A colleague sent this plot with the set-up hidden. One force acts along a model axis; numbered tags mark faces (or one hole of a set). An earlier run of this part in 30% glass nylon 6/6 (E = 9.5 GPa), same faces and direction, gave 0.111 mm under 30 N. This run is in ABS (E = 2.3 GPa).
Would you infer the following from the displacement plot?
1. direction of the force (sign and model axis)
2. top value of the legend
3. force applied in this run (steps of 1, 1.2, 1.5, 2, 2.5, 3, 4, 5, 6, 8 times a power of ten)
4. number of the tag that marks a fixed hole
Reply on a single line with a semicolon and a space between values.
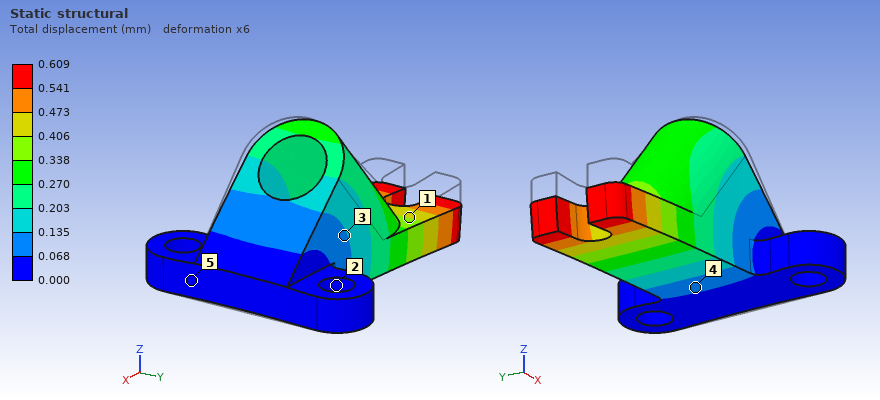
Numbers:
-Z; 0.609 mm; 40 N; 2
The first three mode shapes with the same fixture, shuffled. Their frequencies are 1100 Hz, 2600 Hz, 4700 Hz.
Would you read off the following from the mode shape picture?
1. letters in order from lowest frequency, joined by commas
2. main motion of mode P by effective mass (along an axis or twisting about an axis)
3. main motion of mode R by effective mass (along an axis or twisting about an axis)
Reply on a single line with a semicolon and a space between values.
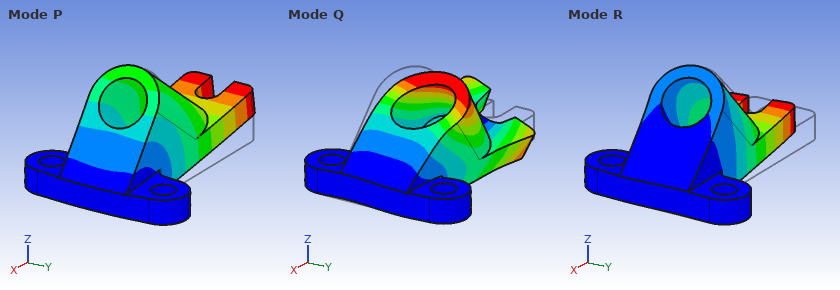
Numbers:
P, R, Q; along Z; along Y
